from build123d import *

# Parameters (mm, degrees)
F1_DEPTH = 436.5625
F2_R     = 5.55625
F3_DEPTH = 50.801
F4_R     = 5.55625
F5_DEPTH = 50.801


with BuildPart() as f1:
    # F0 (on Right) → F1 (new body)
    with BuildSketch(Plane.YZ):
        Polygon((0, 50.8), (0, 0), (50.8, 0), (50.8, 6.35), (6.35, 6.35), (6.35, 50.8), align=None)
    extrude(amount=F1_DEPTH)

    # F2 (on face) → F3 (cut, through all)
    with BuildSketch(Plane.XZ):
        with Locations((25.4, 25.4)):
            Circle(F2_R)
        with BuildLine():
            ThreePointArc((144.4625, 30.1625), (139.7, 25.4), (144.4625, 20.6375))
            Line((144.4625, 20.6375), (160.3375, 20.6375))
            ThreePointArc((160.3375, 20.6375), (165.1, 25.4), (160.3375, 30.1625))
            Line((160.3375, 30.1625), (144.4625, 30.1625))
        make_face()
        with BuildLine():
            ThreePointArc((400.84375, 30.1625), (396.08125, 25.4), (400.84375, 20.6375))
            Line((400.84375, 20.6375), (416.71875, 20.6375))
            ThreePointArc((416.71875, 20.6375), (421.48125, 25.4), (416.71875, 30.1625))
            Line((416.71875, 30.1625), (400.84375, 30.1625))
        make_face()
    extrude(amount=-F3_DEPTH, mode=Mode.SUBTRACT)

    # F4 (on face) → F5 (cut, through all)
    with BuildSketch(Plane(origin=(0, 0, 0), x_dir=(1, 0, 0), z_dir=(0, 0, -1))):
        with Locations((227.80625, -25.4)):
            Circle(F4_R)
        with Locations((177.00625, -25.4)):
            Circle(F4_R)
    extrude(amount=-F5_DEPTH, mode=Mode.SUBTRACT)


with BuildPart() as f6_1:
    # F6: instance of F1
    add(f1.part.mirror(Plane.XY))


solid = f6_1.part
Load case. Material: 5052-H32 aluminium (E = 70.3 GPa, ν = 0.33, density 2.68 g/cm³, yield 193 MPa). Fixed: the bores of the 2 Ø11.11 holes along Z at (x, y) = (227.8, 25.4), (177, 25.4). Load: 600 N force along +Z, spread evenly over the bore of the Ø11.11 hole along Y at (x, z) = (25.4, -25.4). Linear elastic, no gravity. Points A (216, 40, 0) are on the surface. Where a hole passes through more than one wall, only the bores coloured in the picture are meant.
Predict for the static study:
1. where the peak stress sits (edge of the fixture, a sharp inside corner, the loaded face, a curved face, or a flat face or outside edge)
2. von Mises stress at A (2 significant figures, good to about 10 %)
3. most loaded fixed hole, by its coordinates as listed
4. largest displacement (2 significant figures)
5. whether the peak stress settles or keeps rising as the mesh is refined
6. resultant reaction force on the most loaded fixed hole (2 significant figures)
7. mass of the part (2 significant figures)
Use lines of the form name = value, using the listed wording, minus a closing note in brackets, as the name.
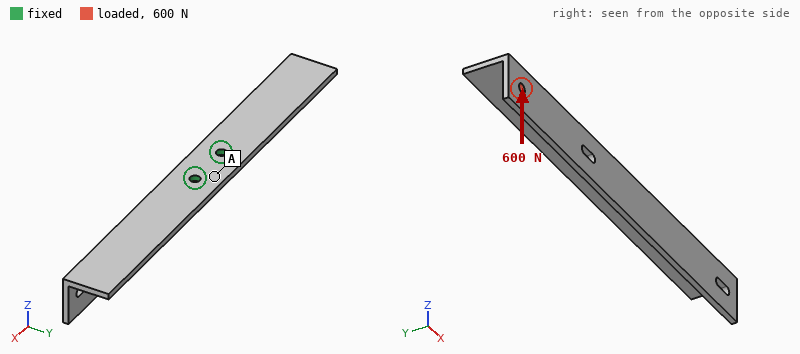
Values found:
where the peak stress sits = edge of the fixture
von Mises stress at A = 8.0 MPa
most loaded fixed hole, by its coordinates as listed = (177, 25.4)
largest displacement = 0.59 mm
whether the peak stress settles or keeps rising as the mesh is refined = keeps rising
resultant reaction force on the most loaded fixed hole = 2.0 kN
mass of the part = 700 g
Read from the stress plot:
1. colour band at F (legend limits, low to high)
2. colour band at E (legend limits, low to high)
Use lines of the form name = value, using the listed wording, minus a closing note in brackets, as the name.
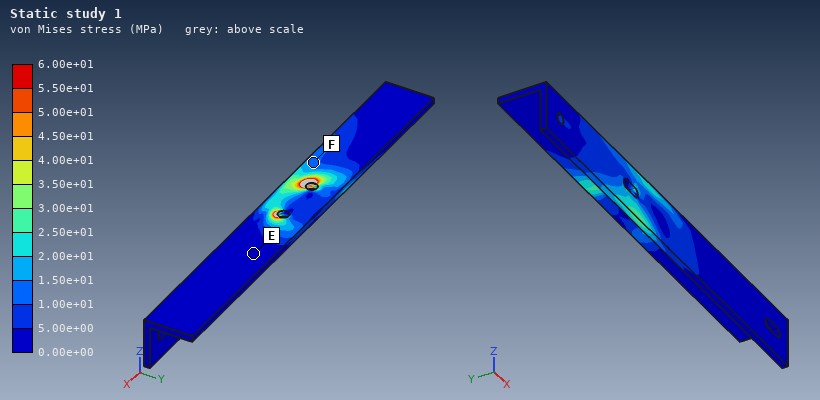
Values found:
colour band at F = 1.00e+01 to 1.50e+01 MPa
colour band at E = 0.00e+00 to 5.00e+00 MPa
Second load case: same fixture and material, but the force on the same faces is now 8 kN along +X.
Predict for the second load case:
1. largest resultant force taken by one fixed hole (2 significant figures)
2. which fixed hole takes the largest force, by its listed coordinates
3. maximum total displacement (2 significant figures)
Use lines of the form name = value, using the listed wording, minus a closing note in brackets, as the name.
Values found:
largest resultant force taken by one fixed hole = 6.0 kN
which fixed hole takes the largest force, by its listed coordinates = (177, 25.4)
maximum total displacement = 0.71 mm
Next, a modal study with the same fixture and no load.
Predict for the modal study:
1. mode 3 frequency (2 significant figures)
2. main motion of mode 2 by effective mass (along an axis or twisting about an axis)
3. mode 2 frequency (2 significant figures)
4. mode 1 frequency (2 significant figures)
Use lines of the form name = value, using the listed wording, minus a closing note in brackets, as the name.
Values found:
mode 3 frequency = 580 Hz
main motion of mode 2 by effective mass = along Y
mode 2 frequency = 490 Hz
mode 1 frequency = 360 Hz
